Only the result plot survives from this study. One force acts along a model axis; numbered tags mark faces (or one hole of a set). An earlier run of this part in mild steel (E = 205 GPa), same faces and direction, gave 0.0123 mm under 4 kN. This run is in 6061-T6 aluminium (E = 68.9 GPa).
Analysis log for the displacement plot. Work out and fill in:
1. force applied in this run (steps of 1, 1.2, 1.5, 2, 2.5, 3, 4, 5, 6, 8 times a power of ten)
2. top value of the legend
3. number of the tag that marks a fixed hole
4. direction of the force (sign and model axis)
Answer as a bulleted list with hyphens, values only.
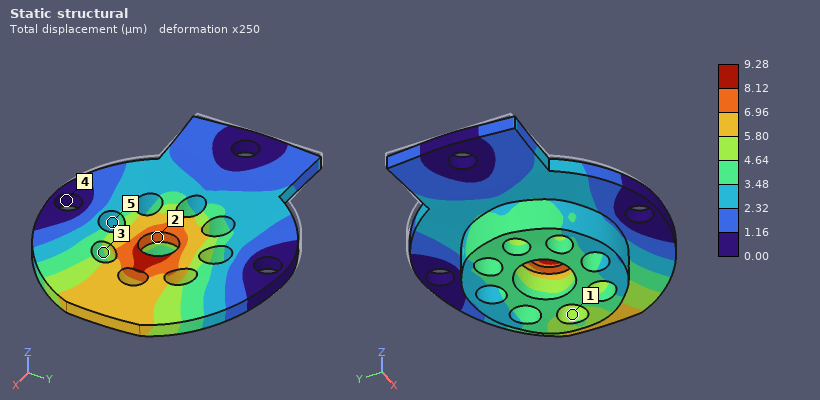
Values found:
- 1 kN
- 9.28 µm
- 4
- +X
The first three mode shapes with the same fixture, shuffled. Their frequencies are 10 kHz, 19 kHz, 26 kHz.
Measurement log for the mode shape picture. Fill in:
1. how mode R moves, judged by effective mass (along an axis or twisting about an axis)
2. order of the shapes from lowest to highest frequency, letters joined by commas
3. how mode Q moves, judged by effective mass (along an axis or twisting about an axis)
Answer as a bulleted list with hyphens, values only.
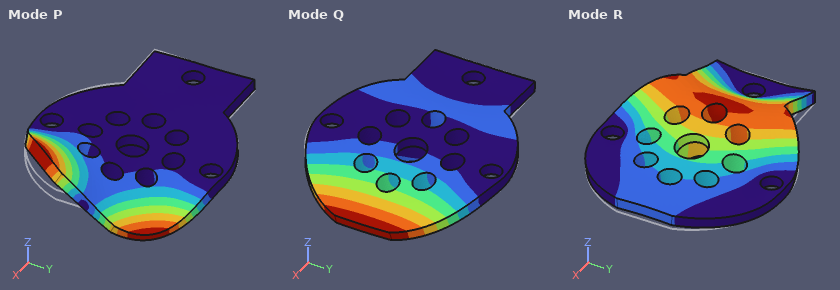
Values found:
- along Z
- Q, R, P
- along Z
